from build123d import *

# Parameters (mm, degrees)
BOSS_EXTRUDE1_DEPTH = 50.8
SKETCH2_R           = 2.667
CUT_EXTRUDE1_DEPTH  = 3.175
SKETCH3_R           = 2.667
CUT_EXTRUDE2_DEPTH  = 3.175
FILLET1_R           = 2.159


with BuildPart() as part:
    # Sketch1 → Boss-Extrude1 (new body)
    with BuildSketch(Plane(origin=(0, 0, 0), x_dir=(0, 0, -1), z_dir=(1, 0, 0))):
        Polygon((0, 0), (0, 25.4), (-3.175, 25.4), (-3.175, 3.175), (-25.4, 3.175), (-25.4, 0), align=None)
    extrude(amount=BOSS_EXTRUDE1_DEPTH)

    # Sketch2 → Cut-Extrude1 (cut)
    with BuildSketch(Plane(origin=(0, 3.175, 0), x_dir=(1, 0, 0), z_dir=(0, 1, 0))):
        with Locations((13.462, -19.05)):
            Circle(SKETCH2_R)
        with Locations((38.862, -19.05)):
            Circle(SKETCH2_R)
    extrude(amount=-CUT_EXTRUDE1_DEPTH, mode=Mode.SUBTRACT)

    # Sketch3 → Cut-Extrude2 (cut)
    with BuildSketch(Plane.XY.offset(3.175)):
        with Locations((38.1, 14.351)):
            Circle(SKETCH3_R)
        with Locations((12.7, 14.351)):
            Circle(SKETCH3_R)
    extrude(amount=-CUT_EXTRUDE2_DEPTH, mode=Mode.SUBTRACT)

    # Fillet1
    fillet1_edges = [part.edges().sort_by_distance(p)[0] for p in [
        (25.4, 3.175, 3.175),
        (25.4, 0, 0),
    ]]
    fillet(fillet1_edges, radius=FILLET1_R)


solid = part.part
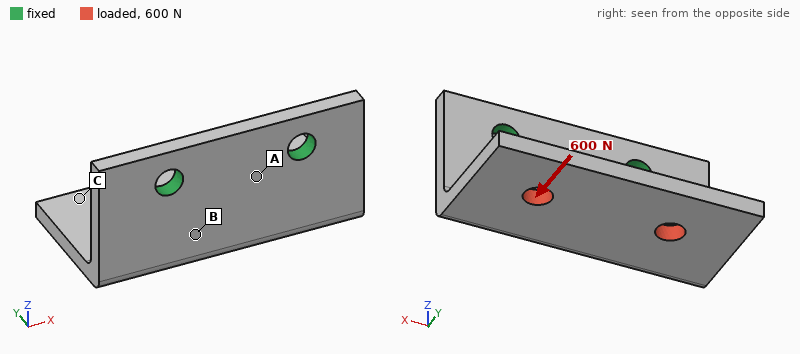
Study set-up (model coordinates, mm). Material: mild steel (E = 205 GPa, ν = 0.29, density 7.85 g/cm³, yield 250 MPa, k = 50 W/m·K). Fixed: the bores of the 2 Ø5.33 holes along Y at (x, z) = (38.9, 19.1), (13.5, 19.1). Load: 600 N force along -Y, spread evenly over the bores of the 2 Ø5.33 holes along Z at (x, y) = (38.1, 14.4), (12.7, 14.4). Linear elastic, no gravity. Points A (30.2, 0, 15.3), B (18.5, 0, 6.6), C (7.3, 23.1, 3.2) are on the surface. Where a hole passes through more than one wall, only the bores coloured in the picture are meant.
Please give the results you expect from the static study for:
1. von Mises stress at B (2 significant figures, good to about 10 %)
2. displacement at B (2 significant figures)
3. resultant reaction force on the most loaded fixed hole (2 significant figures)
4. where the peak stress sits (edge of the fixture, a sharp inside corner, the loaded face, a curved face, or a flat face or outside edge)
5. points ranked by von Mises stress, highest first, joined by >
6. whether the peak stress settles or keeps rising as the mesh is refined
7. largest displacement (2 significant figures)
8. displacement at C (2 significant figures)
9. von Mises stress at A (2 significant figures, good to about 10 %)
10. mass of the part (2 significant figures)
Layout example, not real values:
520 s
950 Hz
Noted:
33 MPa
22 µm
310 N
edge of the fixture
A > B > C
keeps rising
83 µm
73 µm
60 MPa
58 g
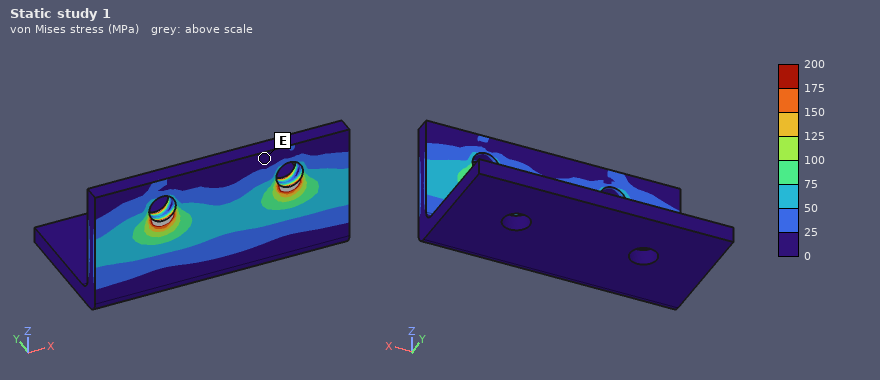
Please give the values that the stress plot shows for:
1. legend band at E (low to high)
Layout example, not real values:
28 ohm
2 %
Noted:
0 to 25 MPa
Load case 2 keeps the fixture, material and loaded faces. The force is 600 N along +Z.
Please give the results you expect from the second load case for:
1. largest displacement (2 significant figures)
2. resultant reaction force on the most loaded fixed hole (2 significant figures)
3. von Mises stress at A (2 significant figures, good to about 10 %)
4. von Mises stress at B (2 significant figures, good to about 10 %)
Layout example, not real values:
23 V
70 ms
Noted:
0.13 mm
320 N
59 MPa
79 MPa
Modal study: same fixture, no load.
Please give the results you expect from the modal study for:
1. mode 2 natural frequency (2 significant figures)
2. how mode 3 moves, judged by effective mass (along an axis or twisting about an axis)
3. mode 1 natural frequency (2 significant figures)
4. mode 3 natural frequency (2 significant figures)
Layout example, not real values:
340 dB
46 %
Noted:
3600 Hz
along Y
2200 Hz
6300 Hz
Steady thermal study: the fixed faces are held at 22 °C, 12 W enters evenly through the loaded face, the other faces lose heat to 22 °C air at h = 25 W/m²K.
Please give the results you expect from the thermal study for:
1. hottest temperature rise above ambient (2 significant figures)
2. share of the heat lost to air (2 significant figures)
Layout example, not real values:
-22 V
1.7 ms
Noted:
42 K
22 %
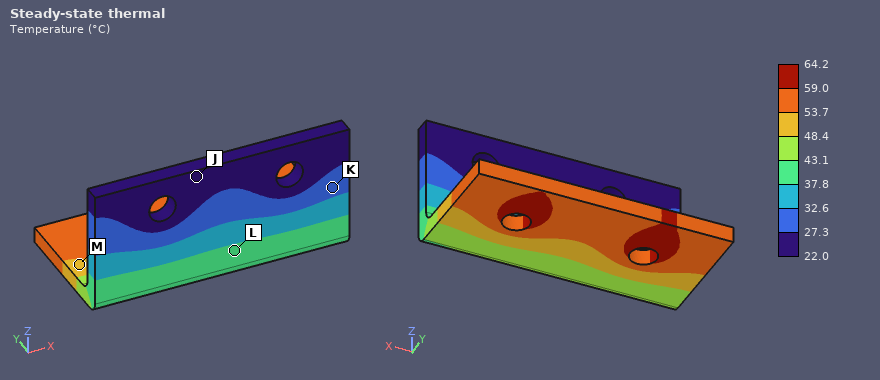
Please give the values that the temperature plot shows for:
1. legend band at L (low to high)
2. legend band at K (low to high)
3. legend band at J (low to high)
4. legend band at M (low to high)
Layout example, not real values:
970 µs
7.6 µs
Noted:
37.8 to 43.1 °C
27.3 to 32.6 °C
22.0 to 27.3 °C
48.4 to 53.7 °C
